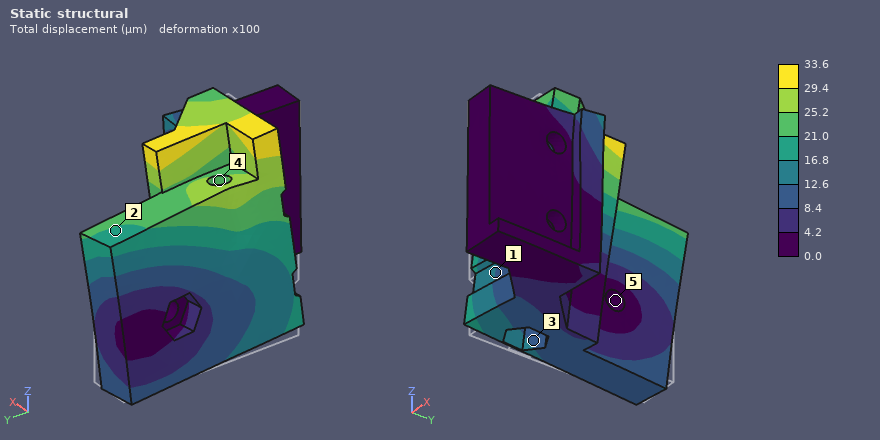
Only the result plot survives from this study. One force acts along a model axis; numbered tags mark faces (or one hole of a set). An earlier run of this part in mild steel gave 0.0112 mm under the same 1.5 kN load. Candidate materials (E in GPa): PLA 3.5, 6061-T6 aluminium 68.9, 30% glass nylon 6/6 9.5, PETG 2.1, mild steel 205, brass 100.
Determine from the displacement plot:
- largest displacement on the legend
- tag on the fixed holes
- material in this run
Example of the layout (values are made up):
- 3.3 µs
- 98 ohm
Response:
- 33.6 µm
- 5
- 6061-T6 aluminium
